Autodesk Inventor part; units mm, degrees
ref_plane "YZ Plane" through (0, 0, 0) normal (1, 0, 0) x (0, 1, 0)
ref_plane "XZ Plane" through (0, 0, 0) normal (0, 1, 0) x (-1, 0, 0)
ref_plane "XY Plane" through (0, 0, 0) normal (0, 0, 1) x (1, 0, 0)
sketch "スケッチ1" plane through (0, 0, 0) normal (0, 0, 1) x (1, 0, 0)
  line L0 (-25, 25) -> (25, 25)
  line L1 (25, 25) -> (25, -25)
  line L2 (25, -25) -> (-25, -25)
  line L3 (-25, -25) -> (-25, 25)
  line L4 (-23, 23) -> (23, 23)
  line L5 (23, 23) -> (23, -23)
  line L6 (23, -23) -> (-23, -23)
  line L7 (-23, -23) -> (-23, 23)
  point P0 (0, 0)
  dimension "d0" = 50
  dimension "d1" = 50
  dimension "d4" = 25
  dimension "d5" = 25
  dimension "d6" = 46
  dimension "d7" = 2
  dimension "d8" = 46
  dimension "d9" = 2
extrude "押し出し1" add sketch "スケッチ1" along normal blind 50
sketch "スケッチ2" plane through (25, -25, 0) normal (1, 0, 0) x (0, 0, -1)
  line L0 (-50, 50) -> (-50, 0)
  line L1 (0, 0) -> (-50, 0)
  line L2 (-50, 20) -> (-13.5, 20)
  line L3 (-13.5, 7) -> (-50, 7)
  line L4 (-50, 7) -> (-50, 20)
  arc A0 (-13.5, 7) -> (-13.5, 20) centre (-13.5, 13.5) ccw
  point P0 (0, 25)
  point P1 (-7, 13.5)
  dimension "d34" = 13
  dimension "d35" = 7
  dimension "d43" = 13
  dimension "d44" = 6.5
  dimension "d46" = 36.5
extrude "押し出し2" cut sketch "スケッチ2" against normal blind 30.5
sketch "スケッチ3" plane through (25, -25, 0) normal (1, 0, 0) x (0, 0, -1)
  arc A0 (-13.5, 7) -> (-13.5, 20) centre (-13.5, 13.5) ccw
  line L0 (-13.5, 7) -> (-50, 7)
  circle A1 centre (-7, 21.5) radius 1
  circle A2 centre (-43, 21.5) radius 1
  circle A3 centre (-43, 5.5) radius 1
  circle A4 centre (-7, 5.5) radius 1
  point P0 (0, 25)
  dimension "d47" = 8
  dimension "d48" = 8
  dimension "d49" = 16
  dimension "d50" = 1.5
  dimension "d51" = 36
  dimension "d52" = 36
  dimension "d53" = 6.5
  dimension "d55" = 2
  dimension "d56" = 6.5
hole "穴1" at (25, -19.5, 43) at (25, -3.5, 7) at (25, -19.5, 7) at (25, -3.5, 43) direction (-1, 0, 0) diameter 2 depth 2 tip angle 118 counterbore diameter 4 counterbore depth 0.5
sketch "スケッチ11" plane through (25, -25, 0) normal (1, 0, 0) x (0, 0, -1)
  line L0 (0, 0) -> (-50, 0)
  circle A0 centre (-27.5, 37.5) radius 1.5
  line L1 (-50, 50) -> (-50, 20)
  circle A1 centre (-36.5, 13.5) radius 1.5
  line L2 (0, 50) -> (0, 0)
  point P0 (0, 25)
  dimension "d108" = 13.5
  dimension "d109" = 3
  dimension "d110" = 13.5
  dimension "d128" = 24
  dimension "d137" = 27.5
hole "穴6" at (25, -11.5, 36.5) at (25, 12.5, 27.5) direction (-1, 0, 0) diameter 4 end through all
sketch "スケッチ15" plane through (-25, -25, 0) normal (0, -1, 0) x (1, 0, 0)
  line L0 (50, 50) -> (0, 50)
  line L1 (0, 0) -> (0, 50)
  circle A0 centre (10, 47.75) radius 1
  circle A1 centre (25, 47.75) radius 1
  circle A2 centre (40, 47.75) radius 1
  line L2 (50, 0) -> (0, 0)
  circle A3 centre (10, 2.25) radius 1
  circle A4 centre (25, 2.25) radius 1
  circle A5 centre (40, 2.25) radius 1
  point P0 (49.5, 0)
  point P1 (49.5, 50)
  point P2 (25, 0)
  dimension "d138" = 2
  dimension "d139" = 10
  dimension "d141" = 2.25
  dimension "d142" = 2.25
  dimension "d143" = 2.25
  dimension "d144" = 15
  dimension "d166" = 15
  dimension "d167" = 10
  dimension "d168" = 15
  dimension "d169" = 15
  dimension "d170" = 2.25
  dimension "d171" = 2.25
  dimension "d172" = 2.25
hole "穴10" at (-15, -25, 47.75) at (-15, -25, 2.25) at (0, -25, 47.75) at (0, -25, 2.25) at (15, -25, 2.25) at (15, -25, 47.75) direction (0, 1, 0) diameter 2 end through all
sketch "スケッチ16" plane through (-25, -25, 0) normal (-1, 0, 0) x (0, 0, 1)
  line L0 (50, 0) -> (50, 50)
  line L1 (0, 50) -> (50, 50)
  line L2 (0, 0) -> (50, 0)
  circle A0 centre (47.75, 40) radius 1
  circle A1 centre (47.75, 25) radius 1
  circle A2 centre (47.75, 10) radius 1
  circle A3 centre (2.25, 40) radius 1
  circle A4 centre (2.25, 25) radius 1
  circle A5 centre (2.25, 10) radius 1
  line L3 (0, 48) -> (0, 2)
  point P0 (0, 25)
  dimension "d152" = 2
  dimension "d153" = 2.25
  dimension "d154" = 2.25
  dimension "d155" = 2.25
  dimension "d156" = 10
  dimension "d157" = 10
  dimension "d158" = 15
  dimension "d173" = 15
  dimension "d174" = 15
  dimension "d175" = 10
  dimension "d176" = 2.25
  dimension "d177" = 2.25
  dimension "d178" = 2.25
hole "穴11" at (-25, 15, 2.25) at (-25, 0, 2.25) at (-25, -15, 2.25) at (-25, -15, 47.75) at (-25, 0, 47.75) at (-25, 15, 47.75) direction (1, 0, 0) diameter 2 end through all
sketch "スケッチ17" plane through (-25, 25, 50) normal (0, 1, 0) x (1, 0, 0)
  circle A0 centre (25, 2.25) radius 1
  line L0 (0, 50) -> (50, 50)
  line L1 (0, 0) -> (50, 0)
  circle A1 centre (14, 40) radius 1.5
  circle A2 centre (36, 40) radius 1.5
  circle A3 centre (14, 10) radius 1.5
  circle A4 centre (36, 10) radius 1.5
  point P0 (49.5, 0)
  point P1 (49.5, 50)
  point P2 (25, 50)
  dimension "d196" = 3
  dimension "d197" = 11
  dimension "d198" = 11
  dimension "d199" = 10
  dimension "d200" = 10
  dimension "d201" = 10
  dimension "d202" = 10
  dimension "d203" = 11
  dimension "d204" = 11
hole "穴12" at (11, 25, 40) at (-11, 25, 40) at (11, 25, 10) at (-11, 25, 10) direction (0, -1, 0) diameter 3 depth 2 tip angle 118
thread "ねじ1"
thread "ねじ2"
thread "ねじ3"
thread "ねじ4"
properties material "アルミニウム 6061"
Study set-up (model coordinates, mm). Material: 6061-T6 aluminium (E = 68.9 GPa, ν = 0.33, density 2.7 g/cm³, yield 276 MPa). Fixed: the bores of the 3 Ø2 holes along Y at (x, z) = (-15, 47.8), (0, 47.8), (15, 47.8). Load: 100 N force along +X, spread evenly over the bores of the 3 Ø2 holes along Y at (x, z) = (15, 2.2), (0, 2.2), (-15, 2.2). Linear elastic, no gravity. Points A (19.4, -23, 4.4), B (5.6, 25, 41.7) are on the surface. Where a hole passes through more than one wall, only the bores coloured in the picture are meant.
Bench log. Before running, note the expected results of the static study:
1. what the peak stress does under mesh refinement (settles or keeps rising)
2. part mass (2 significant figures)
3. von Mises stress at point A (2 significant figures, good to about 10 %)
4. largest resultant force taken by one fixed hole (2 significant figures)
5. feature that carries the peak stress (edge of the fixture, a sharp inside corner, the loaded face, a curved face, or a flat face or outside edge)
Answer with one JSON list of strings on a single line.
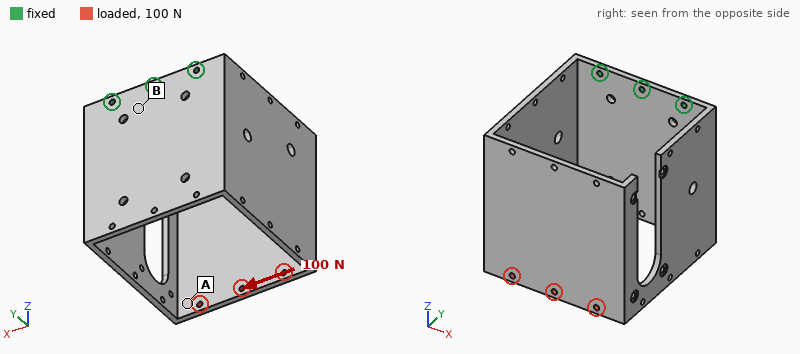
["keeps rising", "48 g", "32 MPa", "190 N", "edge of the fixture"]
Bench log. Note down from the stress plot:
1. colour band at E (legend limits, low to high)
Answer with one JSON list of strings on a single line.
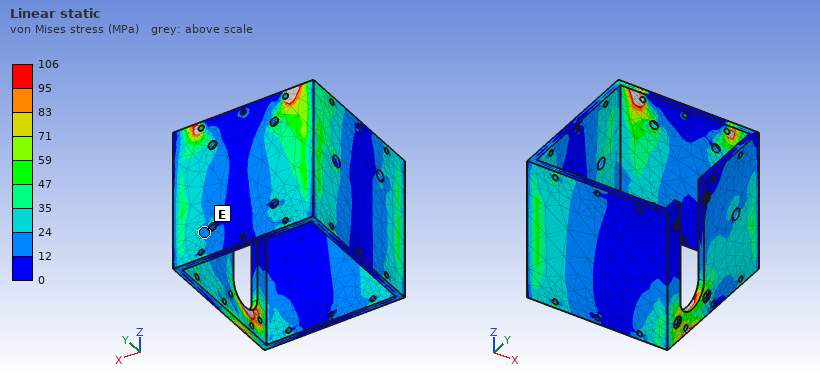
["12 to 24 MPa"]
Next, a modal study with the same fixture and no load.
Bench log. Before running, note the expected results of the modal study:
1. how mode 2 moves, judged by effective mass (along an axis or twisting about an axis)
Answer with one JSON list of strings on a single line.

["along X"]
